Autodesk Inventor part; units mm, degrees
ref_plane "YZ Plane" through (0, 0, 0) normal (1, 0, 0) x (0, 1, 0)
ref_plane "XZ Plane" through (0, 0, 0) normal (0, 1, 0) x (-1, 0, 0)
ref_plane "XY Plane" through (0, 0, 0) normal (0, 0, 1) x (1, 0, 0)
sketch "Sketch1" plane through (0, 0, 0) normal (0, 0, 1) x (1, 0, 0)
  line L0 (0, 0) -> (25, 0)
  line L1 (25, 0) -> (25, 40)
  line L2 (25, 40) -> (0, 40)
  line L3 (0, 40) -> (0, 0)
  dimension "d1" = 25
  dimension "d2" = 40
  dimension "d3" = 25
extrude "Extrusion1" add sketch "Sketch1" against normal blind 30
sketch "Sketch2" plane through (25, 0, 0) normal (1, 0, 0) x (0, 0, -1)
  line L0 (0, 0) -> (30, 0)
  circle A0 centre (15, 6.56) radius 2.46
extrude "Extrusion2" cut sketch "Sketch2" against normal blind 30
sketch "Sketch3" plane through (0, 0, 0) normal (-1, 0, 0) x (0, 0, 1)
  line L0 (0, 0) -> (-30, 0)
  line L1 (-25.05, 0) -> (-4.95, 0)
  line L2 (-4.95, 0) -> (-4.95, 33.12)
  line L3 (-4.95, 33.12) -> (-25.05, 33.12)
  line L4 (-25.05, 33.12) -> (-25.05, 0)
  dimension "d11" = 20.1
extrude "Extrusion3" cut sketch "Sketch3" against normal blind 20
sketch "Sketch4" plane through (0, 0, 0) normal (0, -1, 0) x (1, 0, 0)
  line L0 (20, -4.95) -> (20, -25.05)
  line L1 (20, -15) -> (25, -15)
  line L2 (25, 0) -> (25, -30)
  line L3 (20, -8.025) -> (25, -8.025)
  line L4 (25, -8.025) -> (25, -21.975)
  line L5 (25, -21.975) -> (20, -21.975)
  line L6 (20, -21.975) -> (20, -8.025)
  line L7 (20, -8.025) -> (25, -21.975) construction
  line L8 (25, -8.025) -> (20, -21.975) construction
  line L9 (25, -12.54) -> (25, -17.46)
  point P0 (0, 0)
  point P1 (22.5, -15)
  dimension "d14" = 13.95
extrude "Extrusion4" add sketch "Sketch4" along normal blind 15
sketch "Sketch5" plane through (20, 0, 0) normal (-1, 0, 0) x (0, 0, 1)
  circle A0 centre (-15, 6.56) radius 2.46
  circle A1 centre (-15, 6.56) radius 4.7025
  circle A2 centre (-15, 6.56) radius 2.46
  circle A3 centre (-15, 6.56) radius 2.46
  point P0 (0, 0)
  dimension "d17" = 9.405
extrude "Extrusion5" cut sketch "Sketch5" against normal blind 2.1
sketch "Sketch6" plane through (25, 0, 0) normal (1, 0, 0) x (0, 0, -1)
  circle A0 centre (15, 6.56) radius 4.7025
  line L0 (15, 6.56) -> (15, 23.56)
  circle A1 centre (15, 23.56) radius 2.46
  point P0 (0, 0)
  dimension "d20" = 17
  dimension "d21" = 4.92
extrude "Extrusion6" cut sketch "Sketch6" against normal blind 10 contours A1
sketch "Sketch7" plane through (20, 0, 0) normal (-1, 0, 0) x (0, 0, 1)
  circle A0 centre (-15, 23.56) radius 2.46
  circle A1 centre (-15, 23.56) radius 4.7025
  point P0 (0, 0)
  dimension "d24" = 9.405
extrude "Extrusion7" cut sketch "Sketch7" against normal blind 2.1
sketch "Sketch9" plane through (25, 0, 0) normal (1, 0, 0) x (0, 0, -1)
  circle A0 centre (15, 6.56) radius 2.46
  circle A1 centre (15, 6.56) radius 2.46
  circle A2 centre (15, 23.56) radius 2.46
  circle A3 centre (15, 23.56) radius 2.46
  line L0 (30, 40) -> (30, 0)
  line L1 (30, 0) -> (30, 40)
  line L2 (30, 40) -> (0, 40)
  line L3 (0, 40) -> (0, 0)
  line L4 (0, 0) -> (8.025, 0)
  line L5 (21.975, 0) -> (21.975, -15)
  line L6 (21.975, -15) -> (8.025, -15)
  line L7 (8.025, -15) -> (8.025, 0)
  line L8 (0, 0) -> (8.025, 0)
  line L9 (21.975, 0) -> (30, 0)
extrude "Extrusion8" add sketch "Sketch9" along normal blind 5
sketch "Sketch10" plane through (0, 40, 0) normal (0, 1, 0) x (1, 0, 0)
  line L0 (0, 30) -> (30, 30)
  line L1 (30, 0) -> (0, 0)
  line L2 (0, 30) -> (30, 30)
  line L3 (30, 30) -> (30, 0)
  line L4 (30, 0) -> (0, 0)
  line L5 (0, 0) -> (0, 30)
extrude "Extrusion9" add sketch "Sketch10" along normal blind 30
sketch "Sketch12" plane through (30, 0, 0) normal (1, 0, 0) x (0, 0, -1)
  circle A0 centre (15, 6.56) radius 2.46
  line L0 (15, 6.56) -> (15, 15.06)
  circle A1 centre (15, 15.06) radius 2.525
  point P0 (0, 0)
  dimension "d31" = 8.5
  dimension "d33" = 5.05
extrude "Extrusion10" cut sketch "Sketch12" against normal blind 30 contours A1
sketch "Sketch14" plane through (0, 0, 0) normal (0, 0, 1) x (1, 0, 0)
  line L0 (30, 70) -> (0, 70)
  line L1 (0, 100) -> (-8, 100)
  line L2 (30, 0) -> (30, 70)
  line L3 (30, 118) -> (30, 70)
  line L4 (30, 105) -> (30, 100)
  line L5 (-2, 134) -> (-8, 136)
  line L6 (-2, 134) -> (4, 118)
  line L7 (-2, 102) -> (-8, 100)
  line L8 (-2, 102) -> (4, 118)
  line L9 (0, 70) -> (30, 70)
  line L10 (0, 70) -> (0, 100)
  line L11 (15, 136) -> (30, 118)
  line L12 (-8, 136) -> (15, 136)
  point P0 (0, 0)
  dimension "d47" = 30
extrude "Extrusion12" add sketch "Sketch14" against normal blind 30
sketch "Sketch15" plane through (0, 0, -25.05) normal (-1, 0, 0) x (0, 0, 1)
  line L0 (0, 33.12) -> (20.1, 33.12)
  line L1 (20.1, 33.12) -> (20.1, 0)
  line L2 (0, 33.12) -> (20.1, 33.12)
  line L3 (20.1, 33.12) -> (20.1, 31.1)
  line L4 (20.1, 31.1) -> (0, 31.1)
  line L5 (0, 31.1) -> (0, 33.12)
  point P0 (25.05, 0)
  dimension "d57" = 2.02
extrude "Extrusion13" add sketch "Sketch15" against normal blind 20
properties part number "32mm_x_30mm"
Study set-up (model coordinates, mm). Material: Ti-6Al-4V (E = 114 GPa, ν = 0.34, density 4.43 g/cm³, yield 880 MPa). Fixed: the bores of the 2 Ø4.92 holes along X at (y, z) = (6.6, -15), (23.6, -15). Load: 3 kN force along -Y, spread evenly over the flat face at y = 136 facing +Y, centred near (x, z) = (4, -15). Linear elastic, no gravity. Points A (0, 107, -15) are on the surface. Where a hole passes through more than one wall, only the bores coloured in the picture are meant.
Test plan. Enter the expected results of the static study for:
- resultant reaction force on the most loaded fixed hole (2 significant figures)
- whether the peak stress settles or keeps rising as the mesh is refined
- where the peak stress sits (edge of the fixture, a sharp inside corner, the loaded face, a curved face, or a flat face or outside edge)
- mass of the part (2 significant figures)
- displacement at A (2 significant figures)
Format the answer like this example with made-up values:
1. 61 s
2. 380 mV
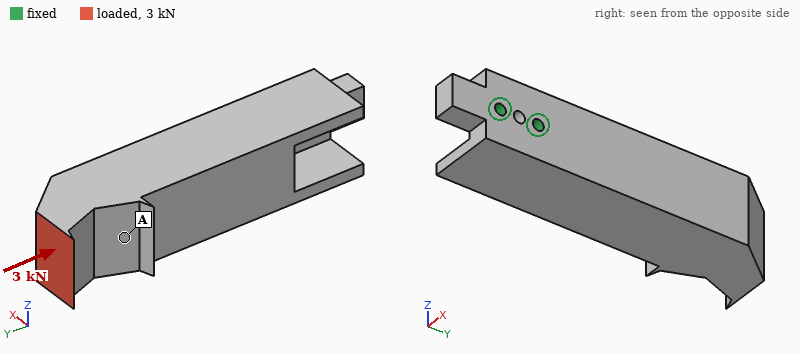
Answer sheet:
1. 3.1 kN
2. keeps rising
3. edge of the fixture
4. 470 g
5. 0.092 mm
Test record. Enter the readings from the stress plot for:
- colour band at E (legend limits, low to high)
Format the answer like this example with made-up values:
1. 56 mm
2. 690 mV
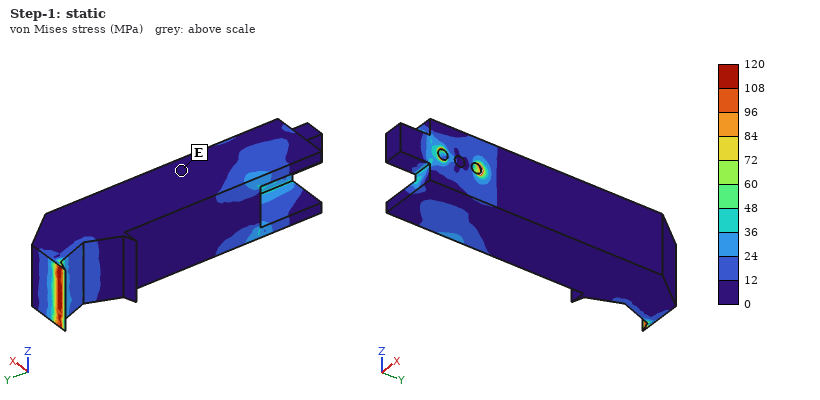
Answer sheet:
1. 0 to 12 MPa
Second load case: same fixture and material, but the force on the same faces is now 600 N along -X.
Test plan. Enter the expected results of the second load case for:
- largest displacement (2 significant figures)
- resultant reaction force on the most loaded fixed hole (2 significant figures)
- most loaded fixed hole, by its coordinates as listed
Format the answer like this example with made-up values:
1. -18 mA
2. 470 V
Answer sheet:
1. 0.14 mm
2. 3.3 kN
3. (23.6, -15)
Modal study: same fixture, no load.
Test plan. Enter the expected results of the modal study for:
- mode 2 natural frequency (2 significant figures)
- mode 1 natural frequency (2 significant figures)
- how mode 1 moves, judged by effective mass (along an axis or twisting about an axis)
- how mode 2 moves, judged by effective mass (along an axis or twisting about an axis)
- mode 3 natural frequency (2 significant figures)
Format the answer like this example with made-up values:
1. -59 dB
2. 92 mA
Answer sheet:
1. 1100 Hz
2. 940 Hz
3. along X
4. along Z
5. 3100 Hz
